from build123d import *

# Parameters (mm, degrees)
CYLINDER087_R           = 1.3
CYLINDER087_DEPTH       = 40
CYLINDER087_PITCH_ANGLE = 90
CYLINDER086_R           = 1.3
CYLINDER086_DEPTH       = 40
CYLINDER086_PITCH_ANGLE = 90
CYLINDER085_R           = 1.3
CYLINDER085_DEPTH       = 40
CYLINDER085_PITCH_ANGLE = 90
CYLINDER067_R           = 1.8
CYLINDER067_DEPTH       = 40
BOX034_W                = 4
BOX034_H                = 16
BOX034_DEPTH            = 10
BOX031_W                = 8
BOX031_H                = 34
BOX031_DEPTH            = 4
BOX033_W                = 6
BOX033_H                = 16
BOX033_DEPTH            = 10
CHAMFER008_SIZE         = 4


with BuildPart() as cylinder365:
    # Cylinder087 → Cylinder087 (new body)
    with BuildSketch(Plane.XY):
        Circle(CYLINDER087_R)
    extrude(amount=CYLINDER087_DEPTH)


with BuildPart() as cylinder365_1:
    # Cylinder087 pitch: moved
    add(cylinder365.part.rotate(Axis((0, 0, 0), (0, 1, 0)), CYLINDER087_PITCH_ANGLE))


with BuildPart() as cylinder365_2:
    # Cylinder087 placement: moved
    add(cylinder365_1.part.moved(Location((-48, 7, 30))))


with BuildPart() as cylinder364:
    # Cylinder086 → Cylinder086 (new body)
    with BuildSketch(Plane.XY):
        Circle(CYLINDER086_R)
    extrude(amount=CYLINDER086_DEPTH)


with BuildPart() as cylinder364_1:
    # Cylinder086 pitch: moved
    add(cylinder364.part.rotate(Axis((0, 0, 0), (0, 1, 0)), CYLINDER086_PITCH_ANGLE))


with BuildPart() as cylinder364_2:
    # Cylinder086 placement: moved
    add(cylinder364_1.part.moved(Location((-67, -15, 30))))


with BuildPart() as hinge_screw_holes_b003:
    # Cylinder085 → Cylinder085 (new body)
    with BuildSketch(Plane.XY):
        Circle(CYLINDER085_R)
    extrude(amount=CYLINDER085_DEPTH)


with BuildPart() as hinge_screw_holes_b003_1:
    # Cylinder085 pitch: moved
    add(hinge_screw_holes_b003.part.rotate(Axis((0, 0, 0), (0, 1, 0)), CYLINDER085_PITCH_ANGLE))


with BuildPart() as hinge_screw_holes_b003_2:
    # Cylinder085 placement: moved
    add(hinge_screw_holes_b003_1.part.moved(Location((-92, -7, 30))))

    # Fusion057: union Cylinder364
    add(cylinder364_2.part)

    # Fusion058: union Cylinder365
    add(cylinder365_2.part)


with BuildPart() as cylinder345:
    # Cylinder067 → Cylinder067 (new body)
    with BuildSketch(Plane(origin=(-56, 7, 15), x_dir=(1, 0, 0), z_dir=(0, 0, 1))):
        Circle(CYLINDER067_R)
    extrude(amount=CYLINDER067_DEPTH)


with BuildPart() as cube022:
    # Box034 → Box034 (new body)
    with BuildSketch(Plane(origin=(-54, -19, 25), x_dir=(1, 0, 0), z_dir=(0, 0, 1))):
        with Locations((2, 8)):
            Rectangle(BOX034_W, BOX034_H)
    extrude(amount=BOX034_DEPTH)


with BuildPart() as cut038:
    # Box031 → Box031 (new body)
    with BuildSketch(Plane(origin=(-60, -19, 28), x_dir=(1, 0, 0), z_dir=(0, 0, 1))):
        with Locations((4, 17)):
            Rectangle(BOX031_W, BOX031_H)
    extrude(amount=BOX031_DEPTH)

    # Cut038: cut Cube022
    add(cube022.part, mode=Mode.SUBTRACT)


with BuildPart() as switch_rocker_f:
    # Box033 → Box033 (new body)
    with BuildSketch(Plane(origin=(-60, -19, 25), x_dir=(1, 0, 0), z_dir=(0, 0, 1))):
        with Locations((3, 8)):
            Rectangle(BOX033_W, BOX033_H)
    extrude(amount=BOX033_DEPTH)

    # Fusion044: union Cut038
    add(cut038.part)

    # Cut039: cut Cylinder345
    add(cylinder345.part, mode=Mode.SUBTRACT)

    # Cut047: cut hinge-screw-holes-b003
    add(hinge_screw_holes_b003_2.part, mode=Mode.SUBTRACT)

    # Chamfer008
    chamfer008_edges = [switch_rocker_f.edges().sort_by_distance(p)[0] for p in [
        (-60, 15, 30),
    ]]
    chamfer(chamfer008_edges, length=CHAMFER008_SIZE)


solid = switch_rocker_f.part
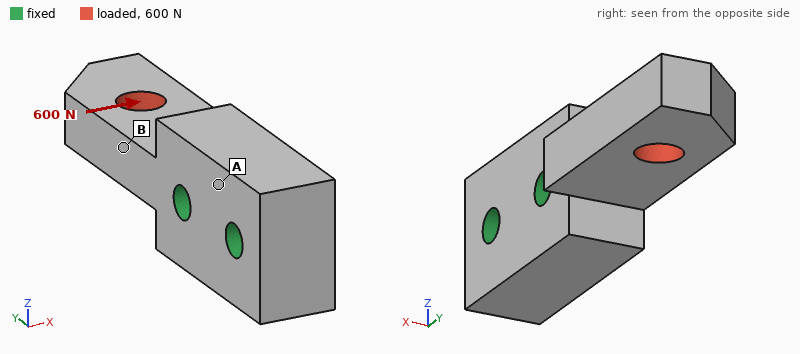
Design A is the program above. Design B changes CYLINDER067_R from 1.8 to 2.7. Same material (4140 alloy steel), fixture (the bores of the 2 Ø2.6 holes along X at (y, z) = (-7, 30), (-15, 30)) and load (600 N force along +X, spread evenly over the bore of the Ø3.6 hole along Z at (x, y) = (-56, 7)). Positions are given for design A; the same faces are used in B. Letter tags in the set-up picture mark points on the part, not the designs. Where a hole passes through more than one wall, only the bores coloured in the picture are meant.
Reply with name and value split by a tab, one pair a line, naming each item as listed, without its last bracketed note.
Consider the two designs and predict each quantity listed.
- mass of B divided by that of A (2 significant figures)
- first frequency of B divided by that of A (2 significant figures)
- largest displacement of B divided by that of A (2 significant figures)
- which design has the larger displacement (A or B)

mass of B divided by that of A	0.96
first frequency of B divided by that of A	1.00
largest displacement of B divided by that of A	1.1
which design has the larger displacement	B
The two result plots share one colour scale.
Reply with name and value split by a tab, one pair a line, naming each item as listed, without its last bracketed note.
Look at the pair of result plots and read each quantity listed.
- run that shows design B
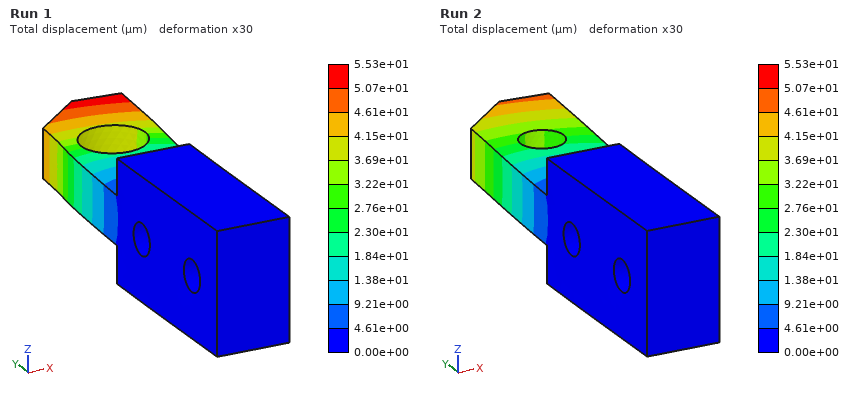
run that shows design B	Run 1
